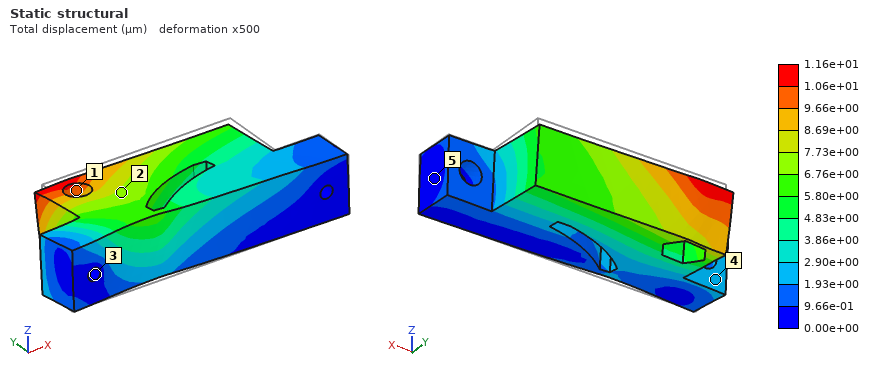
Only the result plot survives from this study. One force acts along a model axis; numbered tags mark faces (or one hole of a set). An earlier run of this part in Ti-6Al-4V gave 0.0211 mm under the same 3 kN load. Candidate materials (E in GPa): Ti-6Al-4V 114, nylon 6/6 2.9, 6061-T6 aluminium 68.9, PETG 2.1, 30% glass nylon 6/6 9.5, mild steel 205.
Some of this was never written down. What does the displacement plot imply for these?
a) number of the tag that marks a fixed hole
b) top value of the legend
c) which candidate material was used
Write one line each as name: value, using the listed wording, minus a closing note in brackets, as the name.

number of the tag that marks a fixed hole: 3
top value of the legend: 1.16e+01 µm
which candidate material was used: mild steel
